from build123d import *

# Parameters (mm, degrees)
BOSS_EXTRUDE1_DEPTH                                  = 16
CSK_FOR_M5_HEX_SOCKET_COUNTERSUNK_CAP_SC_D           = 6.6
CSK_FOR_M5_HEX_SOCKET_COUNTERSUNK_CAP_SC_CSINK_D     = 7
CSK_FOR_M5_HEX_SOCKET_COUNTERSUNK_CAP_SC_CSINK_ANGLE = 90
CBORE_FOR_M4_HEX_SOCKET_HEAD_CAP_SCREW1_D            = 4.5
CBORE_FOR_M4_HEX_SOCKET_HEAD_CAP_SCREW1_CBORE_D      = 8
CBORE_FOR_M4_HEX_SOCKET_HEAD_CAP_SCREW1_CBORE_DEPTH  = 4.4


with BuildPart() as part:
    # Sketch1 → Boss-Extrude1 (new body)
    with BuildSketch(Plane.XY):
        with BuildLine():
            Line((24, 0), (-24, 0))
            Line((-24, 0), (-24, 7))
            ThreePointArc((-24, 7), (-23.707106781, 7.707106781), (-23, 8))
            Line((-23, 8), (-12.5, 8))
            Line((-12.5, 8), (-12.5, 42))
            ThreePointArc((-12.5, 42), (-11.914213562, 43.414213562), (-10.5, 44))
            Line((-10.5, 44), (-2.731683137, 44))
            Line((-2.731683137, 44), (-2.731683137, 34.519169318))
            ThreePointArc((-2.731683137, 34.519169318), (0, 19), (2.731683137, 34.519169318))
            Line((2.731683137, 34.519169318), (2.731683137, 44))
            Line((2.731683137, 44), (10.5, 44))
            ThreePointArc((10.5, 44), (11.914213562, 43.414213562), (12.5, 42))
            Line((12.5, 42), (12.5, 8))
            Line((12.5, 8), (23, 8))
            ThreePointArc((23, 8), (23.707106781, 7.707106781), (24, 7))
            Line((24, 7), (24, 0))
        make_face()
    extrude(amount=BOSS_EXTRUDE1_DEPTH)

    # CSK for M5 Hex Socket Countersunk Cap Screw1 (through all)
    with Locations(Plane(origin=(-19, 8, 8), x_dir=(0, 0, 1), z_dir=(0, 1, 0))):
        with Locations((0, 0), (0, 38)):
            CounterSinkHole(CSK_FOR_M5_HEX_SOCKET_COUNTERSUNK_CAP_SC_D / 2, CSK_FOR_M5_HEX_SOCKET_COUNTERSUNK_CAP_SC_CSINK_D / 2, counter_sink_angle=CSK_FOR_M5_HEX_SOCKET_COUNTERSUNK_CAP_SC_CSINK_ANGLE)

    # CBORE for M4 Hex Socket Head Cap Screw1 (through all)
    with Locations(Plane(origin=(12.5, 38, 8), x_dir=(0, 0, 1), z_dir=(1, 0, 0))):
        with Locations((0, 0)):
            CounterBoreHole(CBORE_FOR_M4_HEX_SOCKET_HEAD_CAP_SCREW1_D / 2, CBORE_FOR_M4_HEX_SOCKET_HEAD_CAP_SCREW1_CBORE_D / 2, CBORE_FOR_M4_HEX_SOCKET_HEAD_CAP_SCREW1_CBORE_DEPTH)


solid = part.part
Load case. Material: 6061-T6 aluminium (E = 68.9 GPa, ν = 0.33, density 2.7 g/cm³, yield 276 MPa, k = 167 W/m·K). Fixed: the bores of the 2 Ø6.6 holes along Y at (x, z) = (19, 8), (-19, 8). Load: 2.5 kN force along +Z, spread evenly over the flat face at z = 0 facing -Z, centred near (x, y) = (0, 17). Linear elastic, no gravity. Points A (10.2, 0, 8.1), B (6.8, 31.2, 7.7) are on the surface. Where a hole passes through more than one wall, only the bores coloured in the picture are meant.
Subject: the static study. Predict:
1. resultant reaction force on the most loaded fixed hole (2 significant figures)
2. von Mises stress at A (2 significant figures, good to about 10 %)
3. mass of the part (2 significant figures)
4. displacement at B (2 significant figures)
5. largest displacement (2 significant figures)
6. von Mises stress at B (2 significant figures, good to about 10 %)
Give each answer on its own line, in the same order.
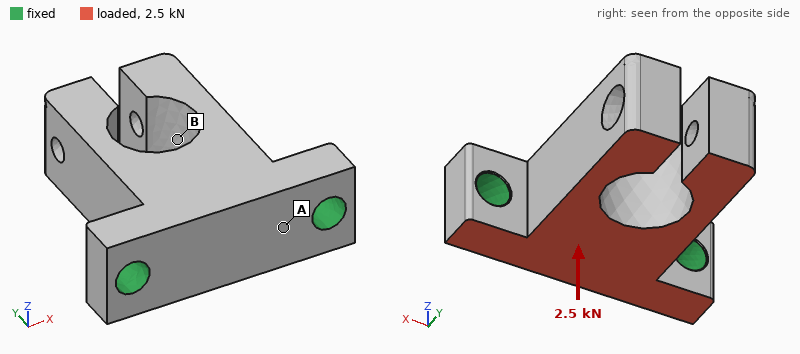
1.3 kN
30 MPa
42 g
0.077 mm
0.12 mm
12 MPa
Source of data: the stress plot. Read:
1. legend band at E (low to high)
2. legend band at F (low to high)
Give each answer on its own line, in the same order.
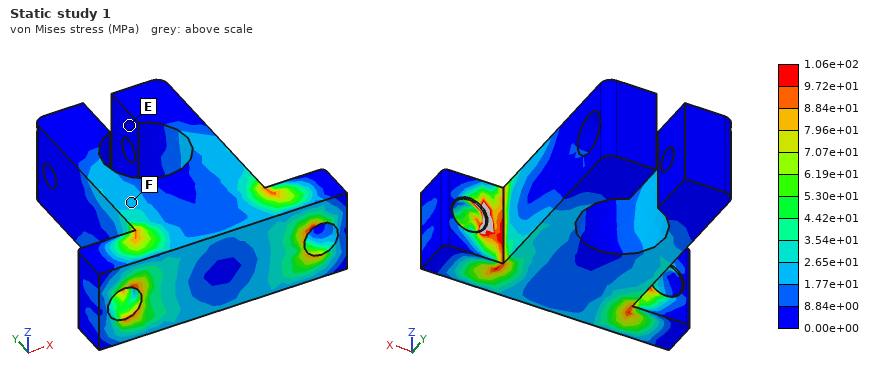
0.00e+00 to 8.84e+00 MPa
1.77e+01 to 2.65e+01 MPa
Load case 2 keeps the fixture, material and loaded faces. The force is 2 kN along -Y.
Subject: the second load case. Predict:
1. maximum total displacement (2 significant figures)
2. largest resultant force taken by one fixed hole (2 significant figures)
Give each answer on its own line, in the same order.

53 µm
1.0 kN
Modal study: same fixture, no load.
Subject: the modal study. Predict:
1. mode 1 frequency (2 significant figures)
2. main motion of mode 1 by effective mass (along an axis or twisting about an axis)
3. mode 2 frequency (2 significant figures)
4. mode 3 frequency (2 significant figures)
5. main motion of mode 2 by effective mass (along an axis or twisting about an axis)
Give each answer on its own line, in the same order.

4400 Hz
along Z
4800 Hz
5000 Hz
along X
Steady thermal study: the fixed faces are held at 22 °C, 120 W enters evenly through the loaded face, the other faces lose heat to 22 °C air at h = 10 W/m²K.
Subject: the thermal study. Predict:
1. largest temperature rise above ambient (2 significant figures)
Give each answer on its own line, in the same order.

57 K
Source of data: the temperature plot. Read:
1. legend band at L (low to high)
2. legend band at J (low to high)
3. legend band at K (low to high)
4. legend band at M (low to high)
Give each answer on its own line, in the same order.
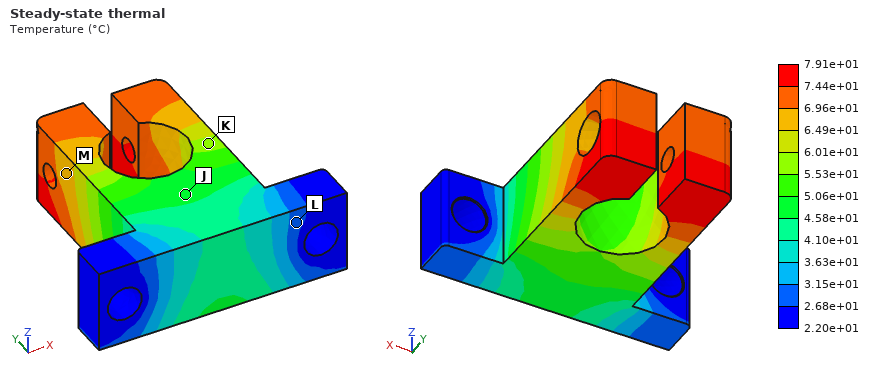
2.68e+01 to 3.15e+01 °C
4.58e+01 to 5.06e+01 °C
5.53e+01 to 6.01e+01 °C
6.49e+01 to 6.96e+01 °C
